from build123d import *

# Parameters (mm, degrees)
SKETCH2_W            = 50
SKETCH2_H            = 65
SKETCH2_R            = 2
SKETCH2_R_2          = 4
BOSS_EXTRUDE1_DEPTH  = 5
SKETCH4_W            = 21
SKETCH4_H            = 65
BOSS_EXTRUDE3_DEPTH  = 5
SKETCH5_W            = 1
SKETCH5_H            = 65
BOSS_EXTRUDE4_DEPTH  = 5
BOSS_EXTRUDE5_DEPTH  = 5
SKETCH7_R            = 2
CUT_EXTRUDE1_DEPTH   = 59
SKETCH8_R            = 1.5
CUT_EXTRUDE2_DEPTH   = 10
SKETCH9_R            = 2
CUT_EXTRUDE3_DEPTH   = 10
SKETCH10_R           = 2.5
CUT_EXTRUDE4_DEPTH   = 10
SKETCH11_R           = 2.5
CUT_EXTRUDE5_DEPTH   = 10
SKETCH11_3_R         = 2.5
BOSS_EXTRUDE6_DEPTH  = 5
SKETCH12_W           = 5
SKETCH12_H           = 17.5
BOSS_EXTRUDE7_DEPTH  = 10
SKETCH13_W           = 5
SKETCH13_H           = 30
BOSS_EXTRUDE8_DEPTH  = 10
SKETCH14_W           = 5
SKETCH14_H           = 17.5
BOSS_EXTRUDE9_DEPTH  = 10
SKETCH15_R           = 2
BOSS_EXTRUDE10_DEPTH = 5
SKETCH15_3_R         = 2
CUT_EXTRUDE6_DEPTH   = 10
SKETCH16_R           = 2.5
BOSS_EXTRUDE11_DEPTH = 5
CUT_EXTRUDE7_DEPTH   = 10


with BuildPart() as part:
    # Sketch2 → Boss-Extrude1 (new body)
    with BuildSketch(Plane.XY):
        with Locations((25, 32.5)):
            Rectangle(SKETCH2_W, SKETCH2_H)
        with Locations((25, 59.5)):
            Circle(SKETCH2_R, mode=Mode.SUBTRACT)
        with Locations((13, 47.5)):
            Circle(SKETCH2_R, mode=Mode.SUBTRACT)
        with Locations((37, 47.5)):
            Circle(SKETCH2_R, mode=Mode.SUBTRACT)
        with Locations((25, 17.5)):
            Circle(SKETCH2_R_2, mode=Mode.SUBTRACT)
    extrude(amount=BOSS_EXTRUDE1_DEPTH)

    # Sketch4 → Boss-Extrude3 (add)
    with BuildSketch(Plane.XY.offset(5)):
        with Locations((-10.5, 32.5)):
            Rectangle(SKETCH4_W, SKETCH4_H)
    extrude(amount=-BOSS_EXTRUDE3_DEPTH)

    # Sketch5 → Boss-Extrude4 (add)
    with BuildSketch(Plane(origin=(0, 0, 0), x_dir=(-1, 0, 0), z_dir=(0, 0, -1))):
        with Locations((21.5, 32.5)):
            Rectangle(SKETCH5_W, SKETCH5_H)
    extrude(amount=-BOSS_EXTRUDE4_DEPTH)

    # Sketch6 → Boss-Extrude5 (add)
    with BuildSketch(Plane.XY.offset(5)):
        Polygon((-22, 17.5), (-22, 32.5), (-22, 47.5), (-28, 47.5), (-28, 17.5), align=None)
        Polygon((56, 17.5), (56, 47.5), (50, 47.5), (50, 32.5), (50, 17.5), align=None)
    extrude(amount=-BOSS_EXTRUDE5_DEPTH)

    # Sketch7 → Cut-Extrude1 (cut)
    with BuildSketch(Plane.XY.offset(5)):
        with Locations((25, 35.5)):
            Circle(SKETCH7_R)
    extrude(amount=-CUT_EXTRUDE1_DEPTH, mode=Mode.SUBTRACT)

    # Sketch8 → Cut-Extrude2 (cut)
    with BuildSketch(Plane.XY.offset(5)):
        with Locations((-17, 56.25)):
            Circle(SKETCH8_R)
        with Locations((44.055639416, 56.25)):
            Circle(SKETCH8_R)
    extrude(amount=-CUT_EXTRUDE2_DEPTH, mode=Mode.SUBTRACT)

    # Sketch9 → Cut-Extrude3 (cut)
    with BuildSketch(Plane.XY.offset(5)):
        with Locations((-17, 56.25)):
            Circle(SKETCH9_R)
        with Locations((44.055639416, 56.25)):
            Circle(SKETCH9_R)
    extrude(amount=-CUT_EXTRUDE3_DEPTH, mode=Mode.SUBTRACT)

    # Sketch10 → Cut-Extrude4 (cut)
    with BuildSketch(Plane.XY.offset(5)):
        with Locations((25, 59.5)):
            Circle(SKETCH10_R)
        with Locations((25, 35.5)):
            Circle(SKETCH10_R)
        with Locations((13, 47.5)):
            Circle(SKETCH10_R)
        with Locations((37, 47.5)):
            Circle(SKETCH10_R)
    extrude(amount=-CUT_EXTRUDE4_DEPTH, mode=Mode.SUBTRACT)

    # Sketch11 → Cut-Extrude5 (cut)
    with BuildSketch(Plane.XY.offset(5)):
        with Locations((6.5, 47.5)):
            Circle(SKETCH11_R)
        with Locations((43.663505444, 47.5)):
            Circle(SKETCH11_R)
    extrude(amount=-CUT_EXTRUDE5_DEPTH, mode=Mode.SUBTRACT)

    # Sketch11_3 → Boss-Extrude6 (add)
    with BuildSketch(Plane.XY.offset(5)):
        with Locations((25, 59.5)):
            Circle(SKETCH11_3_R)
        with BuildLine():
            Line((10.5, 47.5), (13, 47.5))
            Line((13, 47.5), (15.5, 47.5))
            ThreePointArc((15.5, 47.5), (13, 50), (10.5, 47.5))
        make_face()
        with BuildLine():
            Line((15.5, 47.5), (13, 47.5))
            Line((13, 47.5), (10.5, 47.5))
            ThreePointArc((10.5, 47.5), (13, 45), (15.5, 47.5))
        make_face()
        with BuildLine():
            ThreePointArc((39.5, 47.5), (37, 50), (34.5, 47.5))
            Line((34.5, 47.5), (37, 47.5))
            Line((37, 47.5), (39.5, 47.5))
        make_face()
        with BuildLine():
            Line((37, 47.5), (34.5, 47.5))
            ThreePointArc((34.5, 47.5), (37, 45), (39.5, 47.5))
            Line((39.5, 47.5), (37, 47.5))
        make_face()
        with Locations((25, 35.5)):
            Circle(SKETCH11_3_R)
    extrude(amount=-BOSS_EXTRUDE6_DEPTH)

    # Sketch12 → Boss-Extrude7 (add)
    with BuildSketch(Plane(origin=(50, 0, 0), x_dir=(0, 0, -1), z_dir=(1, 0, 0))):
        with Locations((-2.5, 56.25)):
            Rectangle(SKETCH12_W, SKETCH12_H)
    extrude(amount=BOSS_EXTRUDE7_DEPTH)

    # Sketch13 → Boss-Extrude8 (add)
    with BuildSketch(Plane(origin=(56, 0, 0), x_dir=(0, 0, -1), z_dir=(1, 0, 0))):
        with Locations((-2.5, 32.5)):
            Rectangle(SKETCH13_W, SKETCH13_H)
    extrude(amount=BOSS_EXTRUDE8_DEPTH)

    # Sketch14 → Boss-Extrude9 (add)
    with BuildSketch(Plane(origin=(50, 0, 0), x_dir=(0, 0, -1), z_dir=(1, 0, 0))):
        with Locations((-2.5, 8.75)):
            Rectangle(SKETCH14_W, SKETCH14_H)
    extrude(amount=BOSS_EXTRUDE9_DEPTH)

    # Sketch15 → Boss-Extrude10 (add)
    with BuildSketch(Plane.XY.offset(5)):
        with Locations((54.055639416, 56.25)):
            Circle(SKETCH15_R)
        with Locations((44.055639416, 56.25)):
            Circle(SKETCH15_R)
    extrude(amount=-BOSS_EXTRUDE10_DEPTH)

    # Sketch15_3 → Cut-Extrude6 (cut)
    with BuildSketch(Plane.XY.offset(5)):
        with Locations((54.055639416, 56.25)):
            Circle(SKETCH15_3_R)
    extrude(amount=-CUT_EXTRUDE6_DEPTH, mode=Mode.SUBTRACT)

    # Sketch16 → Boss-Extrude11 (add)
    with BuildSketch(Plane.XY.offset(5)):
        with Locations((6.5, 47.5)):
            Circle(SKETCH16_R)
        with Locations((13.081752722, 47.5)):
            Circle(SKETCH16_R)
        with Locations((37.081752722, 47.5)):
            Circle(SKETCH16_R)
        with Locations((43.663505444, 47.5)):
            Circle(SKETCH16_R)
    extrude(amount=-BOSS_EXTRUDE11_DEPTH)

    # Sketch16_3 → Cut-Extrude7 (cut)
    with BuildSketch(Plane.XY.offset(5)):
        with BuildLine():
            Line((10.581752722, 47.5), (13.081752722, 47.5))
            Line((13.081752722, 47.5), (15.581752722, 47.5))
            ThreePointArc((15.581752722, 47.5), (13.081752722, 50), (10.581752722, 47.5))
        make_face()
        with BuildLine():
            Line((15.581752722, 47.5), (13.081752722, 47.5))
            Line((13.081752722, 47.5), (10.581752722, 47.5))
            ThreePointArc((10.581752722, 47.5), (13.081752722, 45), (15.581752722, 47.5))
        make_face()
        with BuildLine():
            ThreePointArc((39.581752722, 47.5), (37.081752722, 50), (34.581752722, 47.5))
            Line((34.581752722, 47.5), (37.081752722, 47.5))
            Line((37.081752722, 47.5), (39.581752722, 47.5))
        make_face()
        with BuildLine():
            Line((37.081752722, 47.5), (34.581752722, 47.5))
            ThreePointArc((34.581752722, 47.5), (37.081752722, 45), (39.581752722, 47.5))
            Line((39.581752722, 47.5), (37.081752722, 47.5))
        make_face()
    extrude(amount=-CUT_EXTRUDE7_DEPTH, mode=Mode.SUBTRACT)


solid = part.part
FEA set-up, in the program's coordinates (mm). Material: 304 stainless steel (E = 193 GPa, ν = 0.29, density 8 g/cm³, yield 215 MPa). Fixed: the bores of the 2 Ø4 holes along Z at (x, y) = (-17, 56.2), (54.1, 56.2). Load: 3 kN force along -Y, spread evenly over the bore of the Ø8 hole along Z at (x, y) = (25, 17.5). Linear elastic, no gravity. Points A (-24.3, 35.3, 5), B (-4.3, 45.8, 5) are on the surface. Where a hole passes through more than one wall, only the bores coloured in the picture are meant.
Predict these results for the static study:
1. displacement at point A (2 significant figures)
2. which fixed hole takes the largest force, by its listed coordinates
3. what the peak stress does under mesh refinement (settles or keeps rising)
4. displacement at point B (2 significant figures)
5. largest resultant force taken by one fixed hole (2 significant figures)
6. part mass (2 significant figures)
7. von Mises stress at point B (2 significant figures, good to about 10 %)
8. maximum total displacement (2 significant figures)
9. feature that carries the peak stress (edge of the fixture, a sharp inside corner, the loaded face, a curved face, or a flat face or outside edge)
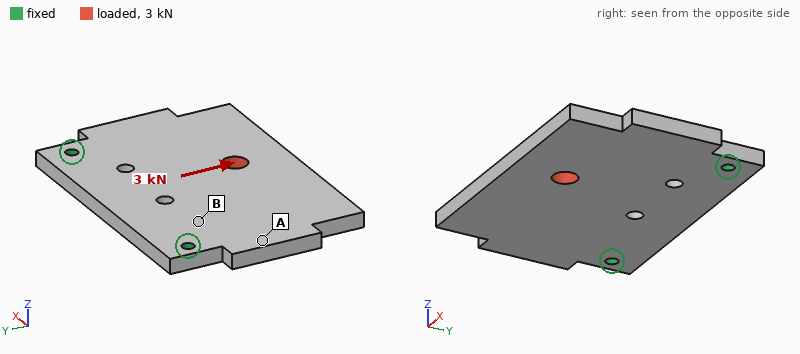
1.0 µm
(54.1, 56.2)
keeps rising
1.9 µm
1.9 kN
220 g
13 MPa
5.8 µm
edge of the fixture
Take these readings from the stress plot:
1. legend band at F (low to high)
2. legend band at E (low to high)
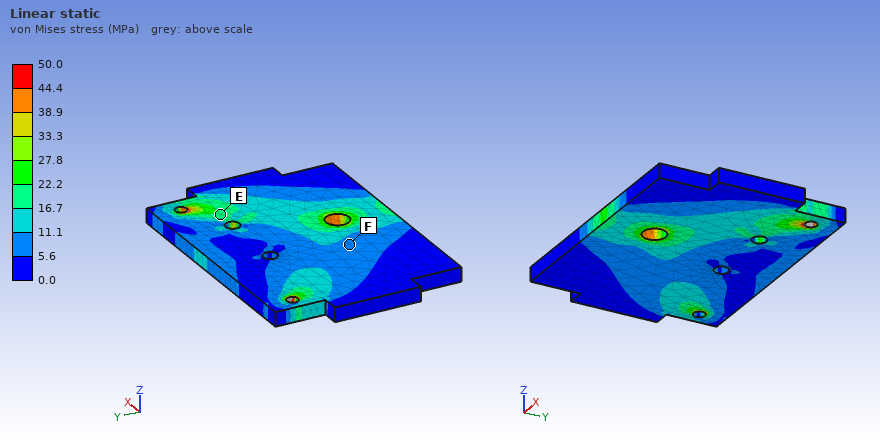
5.6 to 11.1 MPa
16.7 to 22.2 MPa
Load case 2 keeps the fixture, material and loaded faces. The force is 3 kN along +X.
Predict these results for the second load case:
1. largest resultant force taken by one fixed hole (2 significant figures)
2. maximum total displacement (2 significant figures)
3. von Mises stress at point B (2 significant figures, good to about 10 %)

2.2 kN
9.0 µm
19 MPa
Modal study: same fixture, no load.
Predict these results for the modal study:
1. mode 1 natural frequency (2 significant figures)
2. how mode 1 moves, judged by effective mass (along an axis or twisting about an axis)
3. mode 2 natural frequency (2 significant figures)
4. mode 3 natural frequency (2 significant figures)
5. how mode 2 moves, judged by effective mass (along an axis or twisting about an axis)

950 Hz
along Z
2200 Hz
4000 Hz
twisting about Y
